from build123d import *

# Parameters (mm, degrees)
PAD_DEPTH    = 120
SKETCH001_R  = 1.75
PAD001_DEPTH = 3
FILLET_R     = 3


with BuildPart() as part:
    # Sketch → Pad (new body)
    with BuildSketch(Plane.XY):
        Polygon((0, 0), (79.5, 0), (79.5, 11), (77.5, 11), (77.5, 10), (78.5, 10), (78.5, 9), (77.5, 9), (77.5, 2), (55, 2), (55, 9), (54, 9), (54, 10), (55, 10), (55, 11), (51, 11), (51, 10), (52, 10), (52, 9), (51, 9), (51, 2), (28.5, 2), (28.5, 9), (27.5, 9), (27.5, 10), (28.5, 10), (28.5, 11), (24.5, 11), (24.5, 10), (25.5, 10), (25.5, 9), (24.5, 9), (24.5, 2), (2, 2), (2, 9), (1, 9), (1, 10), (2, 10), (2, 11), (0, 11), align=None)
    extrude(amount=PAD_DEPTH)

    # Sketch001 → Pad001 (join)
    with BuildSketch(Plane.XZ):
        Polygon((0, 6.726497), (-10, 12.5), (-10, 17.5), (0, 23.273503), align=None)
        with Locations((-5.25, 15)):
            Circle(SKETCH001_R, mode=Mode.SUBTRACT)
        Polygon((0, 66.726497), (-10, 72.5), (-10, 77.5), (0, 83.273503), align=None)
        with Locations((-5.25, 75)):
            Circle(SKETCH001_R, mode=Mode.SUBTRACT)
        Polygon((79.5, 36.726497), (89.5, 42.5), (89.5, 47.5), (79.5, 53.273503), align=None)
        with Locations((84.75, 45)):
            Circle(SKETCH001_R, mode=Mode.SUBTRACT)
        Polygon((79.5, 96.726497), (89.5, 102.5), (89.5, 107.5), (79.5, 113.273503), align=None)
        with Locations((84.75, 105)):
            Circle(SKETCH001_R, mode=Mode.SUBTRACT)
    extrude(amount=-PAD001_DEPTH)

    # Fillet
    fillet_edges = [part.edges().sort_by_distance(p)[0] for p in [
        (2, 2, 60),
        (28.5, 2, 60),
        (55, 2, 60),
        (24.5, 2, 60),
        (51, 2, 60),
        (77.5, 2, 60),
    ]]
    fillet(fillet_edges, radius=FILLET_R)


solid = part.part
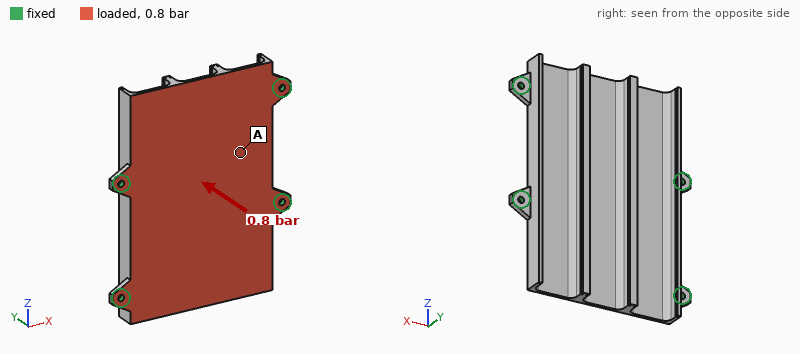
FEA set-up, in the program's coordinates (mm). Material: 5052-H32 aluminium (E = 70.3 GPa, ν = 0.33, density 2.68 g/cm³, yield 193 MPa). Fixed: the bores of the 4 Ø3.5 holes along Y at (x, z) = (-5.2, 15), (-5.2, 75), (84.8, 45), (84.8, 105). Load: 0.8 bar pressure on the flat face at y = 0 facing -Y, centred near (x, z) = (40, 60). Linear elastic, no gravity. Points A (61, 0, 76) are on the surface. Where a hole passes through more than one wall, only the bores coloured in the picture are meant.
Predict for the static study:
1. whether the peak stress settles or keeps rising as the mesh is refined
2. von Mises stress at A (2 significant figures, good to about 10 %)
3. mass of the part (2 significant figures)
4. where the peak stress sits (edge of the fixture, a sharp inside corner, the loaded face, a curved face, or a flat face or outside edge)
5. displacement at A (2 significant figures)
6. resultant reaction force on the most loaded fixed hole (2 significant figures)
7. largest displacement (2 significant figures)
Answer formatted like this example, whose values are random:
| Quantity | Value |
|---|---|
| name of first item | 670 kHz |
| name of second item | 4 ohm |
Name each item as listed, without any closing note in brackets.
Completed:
| Quantity | Value |
|---|---|
| whether the peak stress settles or keeps rising as the mesh is refined | keeps rising |
| von Mises stress at A | 16 MPa |
| mass of the part | 91 g |
| where the peak stress sits | edge of the fixture |
| displacement at A | 0.17 mm |
| resultant reaction force on the most loaded fixed hole | 400 N |
| largest displacement | 0.30 mm |
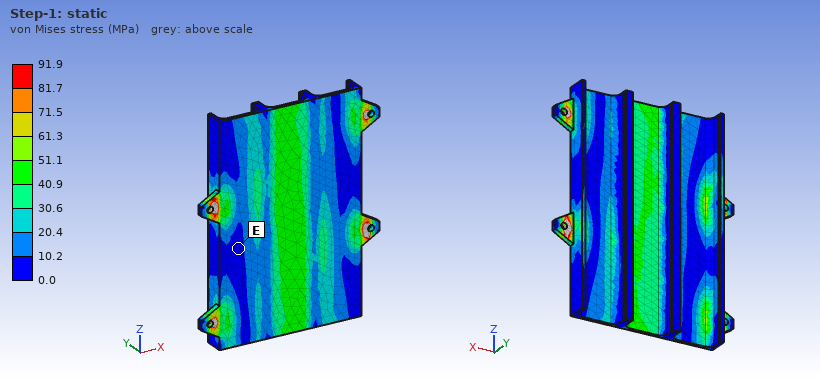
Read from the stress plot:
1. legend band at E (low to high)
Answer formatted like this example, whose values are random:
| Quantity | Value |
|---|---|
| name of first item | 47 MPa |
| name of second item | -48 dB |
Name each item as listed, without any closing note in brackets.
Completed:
| Quantity | Value |
|---|---|
| legend band at E | 0.0 to 10.2 MPa |
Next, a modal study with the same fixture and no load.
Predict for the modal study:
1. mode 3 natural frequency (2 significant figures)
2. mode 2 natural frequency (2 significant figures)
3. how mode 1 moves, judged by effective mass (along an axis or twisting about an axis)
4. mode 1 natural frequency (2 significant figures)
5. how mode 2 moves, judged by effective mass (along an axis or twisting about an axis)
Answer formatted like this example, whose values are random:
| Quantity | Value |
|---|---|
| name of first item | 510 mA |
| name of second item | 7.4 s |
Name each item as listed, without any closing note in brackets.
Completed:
| Quantity | Value |
|---|---|
| mode 3 natural frequency | 2700 Hz |
| mode 2 natural frequency | 1200 Hz |
| how mode 1 moves, judged by effective mass | along Y |
| mode 1 natural frequency | 1000 Hz |
| how mode 2 moves, judged by effective mass | twisting about X |
